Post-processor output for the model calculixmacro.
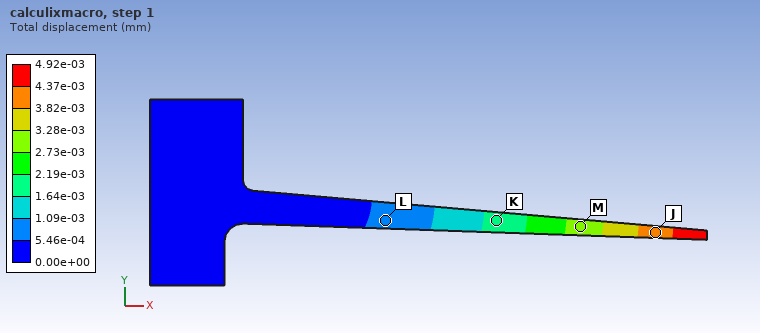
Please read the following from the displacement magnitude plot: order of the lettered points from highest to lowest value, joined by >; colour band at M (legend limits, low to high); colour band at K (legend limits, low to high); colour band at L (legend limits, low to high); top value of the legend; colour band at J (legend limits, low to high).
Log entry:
J > M > K > L
2.73e-03 to 3.28e-03 mm
1.64e-03 to 2.19e-03 mm
5.46e-04 to 1.09e-03 mm
4.92e-03 mm
3.82e-03 to 4.37e-03 mm
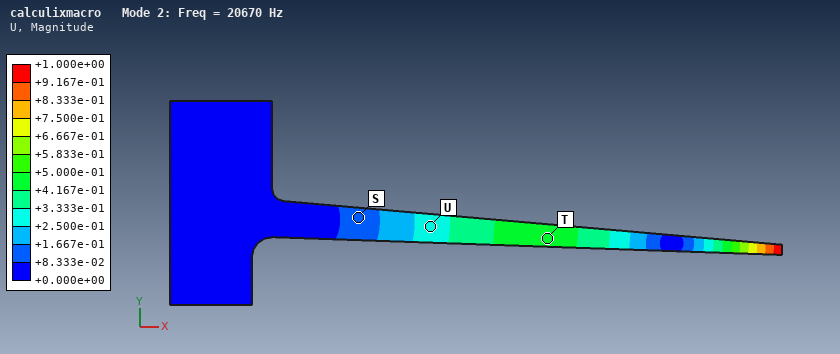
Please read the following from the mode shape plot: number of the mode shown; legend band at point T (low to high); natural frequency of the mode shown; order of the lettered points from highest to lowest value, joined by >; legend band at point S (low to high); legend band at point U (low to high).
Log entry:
2
+4.167e-01 to +5.000e-01
20670 Hz
T > U > S
+8.333e-02 to +1.667e-01
+2.500e-01 to +3.333e-01
